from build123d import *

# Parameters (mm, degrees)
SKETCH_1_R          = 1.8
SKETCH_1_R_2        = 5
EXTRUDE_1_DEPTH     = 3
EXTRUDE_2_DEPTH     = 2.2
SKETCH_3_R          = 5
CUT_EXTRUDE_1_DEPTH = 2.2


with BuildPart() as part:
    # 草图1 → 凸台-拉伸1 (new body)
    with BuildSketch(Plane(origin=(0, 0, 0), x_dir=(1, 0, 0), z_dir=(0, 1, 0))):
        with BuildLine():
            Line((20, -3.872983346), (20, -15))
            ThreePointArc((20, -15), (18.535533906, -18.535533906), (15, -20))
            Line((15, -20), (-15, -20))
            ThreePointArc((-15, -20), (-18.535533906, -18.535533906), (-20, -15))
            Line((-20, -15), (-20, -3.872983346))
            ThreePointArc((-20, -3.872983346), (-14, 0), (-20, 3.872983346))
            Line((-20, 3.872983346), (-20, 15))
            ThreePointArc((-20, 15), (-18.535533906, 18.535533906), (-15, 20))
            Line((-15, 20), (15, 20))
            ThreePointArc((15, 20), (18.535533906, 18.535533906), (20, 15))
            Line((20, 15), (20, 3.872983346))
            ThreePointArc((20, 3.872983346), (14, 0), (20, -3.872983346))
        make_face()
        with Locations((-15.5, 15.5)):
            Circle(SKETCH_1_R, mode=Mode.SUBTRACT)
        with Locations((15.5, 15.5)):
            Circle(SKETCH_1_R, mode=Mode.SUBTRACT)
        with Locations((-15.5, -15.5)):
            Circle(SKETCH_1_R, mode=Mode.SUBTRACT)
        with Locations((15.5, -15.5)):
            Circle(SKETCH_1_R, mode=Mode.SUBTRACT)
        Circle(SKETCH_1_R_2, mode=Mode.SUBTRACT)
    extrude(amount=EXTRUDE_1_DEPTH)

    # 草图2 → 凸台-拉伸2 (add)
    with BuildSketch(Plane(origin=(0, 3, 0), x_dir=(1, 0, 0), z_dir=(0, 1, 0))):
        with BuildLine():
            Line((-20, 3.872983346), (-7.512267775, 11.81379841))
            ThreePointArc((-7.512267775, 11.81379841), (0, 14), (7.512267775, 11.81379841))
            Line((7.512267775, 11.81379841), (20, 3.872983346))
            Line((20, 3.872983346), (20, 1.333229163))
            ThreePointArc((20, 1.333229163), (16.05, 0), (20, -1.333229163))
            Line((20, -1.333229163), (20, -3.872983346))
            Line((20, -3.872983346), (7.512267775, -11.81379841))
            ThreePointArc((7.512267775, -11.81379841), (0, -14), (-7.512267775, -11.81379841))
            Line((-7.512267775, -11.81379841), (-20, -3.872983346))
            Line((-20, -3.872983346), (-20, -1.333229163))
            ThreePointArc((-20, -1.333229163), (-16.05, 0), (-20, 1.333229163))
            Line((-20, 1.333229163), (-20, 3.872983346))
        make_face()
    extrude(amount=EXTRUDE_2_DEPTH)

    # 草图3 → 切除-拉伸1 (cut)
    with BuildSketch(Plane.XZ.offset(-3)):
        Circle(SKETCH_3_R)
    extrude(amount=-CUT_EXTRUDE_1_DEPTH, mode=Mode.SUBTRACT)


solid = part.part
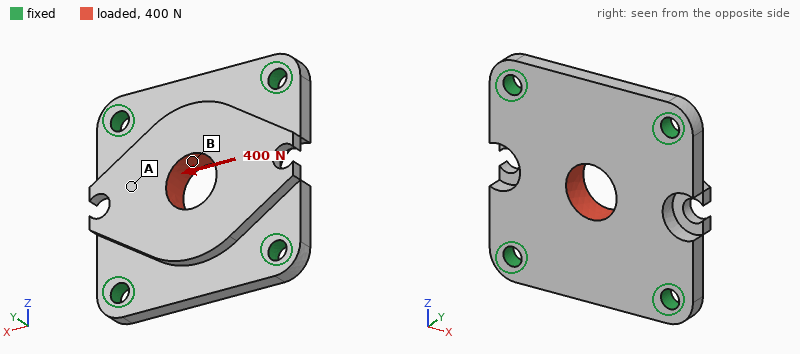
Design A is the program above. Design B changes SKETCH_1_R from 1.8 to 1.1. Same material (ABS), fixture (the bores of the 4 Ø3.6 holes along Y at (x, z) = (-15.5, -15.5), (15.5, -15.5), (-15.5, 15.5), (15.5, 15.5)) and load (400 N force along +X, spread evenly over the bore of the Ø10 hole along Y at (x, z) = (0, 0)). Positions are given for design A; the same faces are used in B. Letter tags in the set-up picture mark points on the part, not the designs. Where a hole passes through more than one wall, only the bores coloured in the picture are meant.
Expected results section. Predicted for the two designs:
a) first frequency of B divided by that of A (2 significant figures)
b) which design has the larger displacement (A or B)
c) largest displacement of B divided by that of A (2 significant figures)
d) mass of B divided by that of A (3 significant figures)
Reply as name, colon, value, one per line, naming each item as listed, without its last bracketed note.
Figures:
first frequency of B divided by that of A: 0.88
which design has the larger displacement: B
largest displacement of B divided by that of A: 1.1
mass of B divided by that of A: 1.01
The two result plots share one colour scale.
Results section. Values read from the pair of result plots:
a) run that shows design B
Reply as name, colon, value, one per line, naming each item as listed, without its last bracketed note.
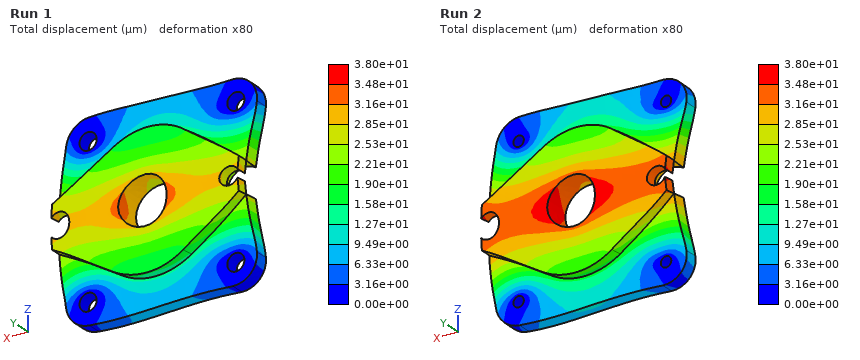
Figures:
run that shows design B: Run 2
